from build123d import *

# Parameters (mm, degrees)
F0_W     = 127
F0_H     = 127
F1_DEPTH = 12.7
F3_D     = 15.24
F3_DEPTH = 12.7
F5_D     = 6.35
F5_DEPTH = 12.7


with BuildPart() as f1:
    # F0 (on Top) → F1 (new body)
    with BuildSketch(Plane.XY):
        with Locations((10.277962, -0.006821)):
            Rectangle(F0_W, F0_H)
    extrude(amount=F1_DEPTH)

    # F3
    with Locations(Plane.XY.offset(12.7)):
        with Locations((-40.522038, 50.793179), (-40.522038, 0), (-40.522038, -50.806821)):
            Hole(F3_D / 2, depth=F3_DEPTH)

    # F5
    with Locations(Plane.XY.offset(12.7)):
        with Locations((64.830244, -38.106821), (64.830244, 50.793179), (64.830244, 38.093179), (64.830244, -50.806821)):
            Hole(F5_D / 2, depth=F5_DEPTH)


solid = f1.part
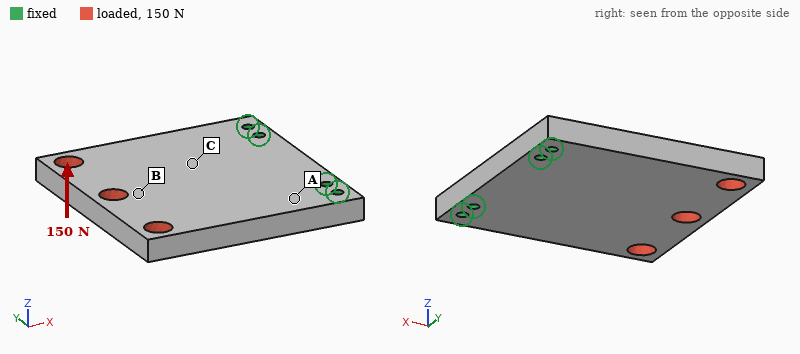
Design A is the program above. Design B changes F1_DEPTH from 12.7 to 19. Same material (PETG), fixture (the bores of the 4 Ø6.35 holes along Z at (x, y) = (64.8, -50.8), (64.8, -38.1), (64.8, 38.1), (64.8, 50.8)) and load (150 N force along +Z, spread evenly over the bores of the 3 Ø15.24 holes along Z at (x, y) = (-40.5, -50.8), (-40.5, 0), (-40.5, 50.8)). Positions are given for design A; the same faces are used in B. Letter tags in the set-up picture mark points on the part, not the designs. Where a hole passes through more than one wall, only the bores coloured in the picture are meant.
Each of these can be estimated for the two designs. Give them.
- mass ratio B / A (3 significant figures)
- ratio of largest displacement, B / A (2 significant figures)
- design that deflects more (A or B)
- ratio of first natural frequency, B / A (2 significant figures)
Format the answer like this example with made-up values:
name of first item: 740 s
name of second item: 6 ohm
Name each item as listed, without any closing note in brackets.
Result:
mass ratio B / A: 1.50
ratio of largest displacement, B / A: 0.32
design that deflects more: A
ratio of first natural frequency, B / A: 1.4
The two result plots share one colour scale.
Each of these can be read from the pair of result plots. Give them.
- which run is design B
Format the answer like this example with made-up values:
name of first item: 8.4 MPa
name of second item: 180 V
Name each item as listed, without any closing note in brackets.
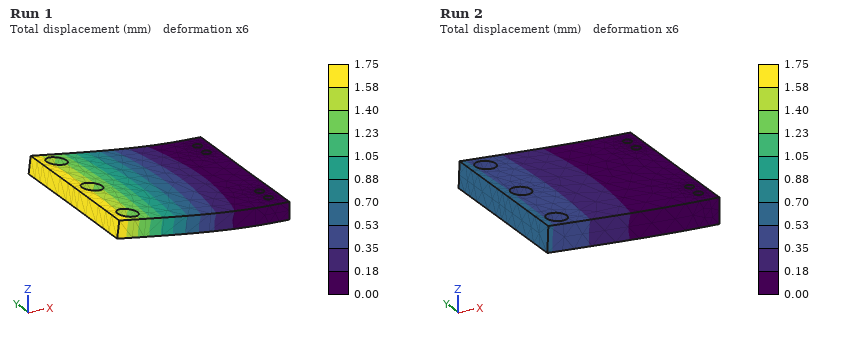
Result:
which run is design B: Run 2
